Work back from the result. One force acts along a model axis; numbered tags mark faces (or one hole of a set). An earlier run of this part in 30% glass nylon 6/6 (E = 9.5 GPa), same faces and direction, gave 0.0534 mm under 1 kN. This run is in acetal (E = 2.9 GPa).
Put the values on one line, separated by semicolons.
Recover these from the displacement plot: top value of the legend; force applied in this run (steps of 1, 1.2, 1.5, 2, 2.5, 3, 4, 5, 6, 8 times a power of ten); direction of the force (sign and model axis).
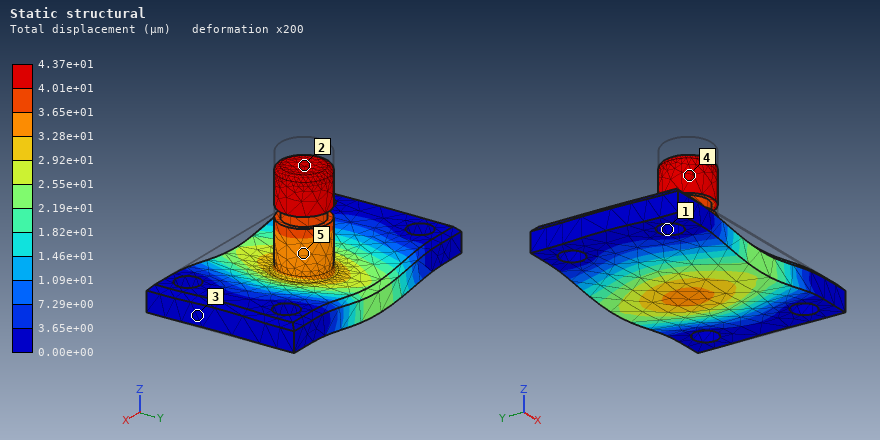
4.37e+01 µm; 250 N; -Z
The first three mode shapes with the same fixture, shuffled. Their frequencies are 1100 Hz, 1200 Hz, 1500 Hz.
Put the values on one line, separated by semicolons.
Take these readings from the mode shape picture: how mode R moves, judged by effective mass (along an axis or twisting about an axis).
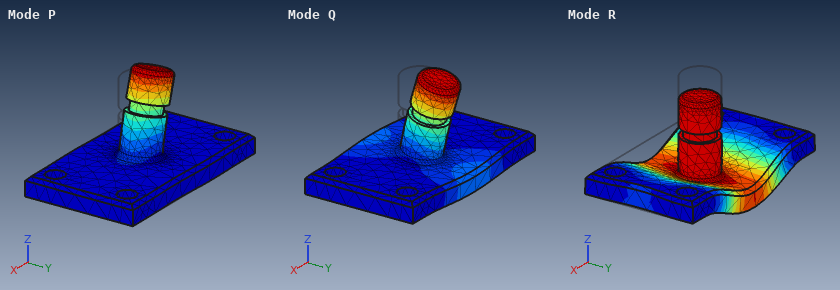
along Z
